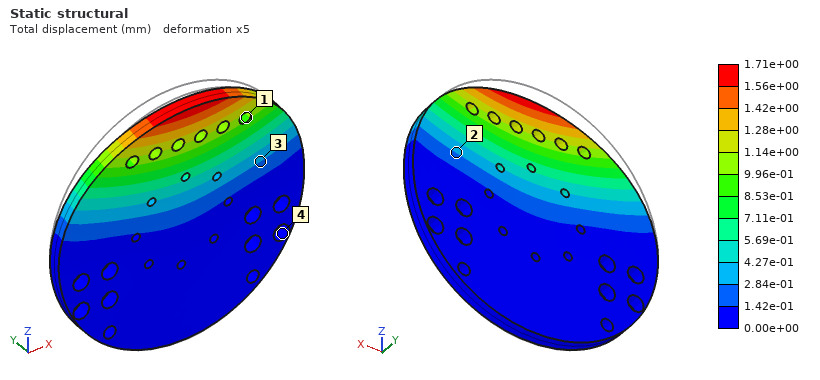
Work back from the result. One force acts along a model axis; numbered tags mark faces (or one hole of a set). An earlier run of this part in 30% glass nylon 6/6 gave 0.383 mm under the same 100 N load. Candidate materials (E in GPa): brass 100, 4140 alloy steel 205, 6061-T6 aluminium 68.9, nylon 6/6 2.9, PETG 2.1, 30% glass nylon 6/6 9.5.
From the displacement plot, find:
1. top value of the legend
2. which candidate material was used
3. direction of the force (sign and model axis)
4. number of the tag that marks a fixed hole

1.71e+00 mm
PETG
-Y
4
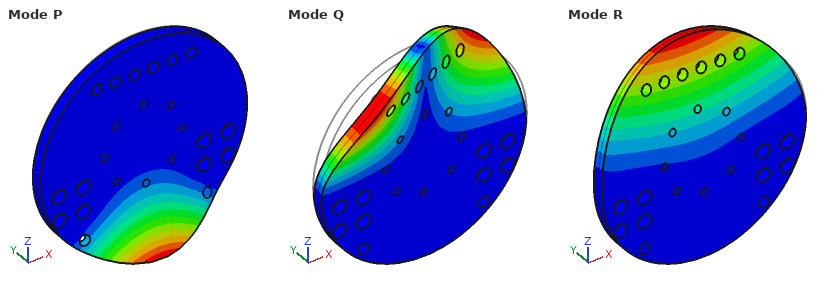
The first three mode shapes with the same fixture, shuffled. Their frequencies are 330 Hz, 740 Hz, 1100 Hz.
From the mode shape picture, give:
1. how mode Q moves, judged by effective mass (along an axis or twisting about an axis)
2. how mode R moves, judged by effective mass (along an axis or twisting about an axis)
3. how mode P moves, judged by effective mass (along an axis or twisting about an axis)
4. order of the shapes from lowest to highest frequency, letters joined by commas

twisting about Z
along Y
along Y
R, Q, P
